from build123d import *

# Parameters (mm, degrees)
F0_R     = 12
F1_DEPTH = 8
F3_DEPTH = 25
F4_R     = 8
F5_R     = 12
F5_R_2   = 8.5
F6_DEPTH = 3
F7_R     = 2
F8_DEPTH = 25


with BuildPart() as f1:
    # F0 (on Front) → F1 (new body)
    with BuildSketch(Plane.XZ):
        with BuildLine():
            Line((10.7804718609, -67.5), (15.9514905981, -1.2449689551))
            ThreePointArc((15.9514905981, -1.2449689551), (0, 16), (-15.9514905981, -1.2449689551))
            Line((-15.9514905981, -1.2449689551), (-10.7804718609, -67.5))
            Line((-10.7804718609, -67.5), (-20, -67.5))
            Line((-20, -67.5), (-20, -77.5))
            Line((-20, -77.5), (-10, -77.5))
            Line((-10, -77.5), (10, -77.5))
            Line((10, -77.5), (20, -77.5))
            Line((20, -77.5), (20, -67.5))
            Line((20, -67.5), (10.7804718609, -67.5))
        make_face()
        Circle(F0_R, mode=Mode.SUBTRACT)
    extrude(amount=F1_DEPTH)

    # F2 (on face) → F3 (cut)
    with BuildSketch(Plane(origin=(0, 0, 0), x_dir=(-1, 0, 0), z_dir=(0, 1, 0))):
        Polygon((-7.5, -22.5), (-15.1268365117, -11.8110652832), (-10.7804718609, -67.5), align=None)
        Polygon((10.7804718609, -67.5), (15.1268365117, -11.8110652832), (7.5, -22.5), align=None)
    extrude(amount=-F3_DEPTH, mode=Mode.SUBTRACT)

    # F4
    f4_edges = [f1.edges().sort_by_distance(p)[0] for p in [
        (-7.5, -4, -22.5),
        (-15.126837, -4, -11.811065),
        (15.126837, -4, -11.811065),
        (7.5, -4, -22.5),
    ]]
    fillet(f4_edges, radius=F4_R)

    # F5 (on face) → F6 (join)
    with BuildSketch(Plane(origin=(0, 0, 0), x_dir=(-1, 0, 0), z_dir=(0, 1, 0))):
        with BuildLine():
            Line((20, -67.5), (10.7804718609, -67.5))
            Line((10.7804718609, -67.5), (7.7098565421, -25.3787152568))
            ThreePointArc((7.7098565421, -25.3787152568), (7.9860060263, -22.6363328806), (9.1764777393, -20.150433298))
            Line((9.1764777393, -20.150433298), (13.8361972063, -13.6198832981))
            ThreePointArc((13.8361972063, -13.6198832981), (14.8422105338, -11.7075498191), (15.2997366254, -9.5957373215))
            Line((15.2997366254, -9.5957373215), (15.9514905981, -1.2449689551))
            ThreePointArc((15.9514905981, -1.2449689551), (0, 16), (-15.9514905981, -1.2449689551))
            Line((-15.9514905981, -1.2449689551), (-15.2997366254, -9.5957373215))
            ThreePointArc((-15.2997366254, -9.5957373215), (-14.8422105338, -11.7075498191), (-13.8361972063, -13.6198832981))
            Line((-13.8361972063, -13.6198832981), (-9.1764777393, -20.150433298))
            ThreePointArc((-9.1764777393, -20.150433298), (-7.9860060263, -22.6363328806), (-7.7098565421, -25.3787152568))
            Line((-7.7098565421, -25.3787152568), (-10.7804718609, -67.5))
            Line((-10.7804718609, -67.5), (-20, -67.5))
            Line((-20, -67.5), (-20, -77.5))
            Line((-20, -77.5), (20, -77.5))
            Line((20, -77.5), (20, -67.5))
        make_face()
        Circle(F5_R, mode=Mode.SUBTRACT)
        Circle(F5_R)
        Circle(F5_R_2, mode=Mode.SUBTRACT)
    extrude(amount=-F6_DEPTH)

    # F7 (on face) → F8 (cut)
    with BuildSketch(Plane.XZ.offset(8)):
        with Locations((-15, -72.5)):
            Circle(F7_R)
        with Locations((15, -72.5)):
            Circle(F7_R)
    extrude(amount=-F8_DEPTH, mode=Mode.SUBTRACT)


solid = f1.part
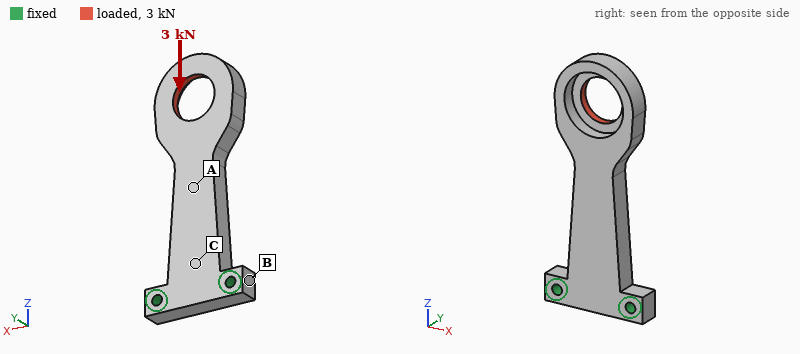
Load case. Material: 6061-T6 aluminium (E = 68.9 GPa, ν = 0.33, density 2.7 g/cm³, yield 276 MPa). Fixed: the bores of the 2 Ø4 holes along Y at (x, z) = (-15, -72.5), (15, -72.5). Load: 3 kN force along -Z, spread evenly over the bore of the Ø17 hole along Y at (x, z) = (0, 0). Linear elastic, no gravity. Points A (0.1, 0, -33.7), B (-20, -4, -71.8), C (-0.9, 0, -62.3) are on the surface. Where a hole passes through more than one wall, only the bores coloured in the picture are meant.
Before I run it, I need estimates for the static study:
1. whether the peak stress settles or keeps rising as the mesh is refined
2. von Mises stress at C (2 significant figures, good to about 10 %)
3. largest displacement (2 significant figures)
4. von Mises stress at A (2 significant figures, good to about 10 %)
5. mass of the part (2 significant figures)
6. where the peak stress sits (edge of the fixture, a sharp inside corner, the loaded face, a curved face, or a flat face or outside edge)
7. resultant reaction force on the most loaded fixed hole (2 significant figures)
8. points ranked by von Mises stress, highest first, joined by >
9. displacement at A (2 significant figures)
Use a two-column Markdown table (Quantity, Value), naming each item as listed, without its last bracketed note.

| Quantity | Value |
|---|---|
| whether the peak stress settles or keeps rising as the mesh is refined | keeps rising |
| von Mises stress at C | 41 MPa |
| largest displacement | 0.58 mm |
| von Mises stress at A | 65 MPa |
| mass of the part | 40 g |
| where the peak stress sits | edge of the fixture |
| resultant reaction force on the most loaded fixed hole | 1.6 kN |
| points ranked by von Mises stress, highest first, joined by > | A > C > B |
| displacement at A | 0.13 mm |
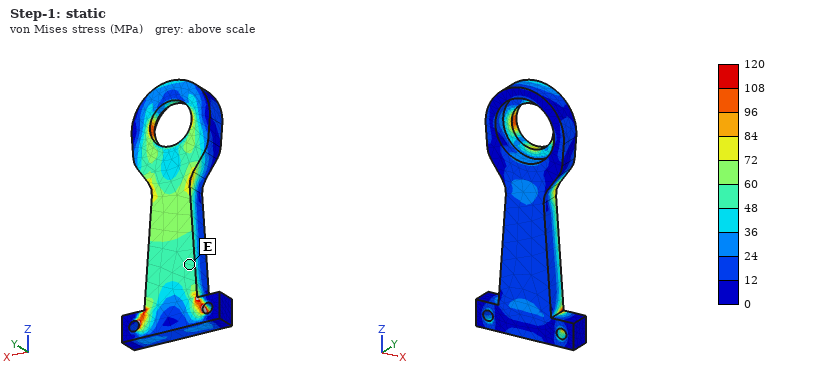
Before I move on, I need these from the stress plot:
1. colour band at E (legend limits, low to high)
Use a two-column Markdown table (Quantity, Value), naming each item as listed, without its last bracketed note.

| Quantity | Value |
|---|---|
| colour band at E | 48 to 60 MPa |
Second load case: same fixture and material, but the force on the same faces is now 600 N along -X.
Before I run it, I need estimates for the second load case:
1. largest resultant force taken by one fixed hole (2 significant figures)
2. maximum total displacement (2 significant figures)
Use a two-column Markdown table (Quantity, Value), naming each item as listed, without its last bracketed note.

| Quantity | Value |
|---|---|
| largest resultant force taken by one fixed hole | 1.7 kN |
| maximum total displacement | 0.36 mm |
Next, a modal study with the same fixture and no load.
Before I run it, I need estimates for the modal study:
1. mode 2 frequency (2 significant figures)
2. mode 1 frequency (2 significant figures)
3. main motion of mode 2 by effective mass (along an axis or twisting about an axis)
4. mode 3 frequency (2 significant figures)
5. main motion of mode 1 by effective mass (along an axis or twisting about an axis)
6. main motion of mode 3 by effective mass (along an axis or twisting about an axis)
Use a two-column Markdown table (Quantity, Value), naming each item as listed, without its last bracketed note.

| Quantity | Value |
|---|---|
| mode 2 frequency | 2100 Hz |
| mode 1 frequency | 830 Hz |
| main motion of mode 2 by effective mass | along X |
| mode 3 frequency | 4200 Hz |
| main motion of mode 1 by effective mass | along Y |
| main motion of mode 3 by effective mass | twisting about Z |
